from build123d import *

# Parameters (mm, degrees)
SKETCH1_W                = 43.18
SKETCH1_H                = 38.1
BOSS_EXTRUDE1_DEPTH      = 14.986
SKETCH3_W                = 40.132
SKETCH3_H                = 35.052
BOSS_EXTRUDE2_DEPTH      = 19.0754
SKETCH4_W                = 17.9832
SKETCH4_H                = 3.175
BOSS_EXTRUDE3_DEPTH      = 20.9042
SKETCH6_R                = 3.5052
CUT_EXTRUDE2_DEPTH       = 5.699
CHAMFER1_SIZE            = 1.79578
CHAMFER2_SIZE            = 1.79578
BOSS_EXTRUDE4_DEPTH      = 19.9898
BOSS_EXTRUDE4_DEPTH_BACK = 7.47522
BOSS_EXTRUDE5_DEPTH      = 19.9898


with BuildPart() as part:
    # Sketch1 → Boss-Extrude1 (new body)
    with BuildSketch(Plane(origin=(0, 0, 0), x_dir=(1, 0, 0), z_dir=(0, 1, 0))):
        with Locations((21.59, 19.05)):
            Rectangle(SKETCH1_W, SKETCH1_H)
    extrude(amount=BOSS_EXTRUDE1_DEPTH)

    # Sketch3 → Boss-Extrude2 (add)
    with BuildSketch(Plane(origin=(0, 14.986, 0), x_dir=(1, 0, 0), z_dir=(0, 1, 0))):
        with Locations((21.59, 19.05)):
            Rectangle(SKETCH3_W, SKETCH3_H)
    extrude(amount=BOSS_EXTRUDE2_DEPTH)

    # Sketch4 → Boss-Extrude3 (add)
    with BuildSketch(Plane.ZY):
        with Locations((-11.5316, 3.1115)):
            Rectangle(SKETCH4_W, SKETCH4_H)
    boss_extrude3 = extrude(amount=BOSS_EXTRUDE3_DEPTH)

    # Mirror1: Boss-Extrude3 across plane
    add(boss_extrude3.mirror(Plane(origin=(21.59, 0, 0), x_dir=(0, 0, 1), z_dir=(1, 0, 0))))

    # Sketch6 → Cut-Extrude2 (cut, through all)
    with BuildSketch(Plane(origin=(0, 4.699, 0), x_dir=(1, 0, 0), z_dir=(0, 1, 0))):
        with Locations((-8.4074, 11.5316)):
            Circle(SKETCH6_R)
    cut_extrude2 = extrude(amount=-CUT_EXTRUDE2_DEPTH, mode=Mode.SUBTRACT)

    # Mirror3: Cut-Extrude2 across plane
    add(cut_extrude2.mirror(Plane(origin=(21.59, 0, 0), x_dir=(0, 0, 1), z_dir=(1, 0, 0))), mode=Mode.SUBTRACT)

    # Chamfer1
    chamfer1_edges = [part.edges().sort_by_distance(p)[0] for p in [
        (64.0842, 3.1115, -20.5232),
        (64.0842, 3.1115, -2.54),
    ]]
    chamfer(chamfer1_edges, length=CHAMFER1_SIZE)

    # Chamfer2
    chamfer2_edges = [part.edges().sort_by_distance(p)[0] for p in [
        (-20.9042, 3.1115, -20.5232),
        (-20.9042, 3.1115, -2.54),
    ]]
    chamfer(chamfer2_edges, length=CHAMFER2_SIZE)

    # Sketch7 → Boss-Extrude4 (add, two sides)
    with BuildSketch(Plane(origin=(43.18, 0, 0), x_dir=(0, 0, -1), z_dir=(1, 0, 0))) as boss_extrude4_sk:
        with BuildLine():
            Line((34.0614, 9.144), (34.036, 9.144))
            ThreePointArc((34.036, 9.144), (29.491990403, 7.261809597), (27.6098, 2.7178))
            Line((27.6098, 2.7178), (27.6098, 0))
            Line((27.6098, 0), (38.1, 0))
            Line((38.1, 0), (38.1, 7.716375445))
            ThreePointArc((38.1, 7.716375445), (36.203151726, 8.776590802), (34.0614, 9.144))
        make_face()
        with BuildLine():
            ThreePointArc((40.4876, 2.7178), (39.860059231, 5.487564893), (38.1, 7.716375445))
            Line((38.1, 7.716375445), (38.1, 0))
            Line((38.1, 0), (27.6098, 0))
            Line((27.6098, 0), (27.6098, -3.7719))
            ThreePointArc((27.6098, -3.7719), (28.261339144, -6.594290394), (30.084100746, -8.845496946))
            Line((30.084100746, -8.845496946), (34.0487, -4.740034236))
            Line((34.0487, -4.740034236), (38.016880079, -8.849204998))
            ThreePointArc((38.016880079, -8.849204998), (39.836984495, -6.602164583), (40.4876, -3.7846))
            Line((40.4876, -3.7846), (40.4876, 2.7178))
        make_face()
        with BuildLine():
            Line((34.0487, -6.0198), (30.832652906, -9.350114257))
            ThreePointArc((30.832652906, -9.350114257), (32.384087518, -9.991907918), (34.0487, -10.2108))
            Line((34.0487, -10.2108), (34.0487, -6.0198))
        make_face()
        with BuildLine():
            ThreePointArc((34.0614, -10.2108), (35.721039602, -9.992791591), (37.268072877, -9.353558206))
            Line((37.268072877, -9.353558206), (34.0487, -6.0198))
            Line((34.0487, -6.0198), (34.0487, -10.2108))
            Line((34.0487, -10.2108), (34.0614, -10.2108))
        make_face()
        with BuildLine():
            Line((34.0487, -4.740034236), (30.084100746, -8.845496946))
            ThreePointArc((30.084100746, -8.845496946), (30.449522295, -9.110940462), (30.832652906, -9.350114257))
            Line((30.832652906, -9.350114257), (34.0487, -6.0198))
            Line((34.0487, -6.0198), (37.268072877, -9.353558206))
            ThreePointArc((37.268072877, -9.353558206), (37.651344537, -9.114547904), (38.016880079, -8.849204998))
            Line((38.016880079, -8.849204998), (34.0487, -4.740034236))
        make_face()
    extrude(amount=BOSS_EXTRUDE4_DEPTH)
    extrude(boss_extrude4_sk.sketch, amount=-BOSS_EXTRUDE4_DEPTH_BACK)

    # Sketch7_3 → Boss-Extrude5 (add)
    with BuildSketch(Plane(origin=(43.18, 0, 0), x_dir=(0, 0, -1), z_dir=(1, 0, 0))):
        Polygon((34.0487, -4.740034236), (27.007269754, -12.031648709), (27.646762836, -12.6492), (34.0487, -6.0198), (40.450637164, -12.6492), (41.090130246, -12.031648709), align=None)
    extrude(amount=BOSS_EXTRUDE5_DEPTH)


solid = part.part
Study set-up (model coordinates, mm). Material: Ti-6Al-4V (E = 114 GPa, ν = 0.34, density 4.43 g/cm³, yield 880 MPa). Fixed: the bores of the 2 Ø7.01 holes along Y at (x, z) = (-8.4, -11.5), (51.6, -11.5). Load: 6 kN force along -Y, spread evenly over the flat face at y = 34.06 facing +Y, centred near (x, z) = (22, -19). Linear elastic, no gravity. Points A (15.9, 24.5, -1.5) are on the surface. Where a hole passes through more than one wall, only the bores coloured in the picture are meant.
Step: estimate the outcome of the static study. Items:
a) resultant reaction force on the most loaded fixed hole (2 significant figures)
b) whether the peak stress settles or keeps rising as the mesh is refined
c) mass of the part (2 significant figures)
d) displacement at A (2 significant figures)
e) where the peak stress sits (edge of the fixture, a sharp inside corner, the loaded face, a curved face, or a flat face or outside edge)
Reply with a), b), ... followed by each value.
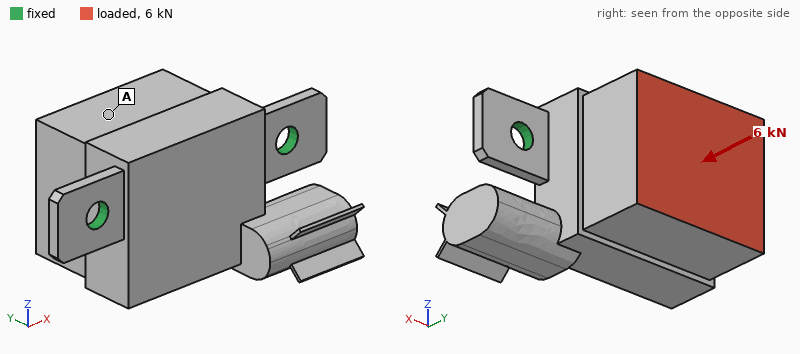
a) 3.2 kN
b) keeps rising
c) 260 g
d) 0.23 mm
e) edge of the fixture
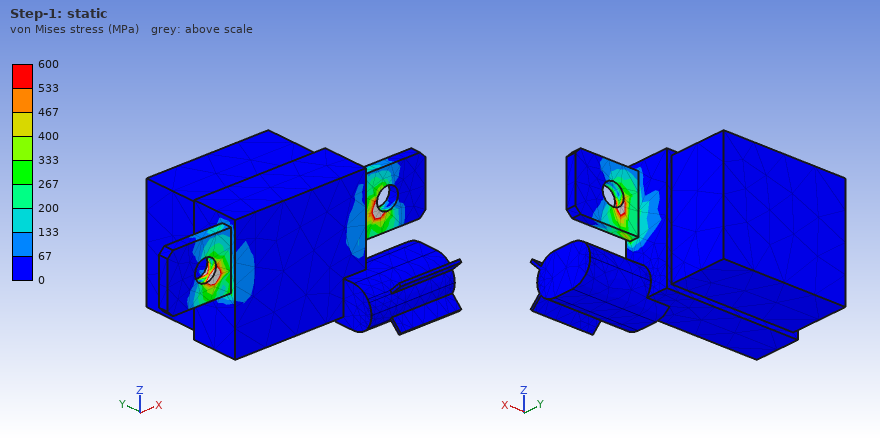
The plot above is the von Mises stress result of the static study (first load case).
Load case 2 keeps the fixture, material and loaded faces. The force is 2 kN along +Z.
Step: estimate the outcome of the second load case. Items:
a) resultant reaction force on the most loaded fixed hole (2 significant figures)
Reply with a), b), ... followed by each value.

a) 1.0 kN
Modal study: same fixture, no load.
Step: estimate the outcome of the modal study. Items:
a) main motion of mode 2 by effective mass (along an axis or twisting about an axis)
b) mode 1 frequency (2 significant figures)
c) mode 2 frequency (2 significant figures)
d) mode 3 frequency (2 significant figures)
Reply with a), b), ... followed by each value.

a) along Y
b) 980 Hz
c) 4500 Hz
d) 5000 Hz
